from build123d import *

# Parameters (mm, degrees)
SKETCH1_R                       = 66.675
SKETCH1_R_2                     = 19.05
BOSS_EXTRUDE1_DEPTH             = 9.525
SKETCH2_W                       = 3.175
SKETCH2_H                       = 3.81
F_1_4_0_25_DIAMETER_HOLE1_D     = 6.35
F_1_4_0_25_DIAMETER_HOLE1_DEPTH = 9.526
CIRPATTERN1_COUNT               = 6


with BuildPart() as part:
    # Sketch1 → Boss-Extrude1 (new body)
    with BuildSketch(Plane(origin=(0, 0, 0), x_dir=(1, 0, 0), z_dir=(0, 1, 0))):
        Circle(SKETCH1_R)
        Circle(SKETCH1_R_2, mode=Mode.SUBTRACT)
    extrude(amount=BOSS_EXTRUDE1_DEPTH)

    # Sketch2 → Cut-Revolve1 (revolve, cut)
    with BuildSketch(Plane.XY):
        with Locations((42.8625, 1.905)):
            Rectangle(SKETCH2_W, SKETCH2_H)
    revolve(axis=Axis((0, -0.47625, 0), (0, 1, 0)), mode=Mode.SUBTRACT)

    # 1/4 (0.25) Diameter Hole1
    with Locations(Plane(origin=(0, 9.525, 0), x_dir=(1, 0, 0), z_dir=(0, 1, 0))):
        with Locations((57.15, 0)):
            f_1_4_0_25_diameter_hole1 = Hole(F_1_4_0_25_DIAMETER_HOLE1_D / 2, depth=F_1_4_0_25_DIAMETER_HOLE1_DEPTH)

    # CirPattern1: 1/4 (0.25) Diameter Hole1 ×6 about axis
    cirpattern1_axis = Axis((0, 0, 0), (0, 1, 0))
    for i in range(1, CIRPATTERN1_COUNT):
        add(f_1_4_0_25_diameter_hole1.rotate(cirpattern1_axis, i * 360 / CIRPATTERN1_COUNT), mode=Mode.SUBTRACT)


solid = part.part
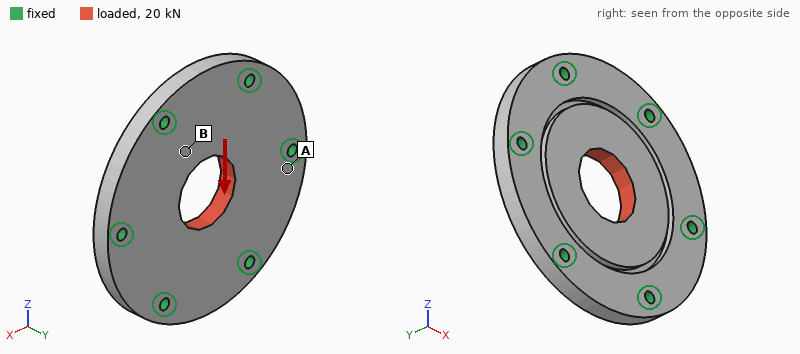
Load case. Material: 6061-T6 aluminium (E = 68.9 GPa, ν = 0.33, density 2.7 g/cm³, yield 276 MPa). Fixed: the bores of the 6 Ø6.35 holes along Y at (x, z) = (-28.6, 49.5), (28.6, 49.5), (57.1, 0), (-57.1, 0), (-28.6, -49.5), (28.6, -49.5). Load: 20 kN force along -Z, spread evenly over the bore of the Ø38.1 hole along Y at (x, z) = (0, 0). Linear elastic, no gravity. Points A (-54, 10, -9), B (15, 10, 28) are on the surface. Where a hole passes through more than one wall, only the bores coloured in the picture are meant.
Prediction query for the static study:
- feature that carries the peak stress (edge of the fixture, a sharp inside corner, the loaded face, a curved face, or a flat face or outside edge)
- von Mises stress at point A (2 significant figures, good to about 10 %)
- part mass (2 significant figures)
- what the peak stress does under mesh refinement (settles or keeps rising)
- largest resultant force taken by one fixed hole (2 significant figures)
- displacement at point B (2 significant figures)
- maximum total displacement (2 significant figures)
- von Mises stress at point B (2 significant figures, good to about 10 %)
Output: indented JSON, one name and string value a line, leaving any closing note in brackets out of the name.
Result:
{
  "feature that carries the peak stress": "edge of the fixture",
  "von Mises stress at point A": "7.9 MPa",
  "part mass": "320 g",
  "what the peak stress does under mesh refinement": "keeps rising",
  "largest resultant force taken by one fixed hole": "4.2 kN",
  "displacement at point B": "8.9 µm",
  "maximum total displacement": "15 µm",
  "von Mises stress at point B": "18 MPa"
}
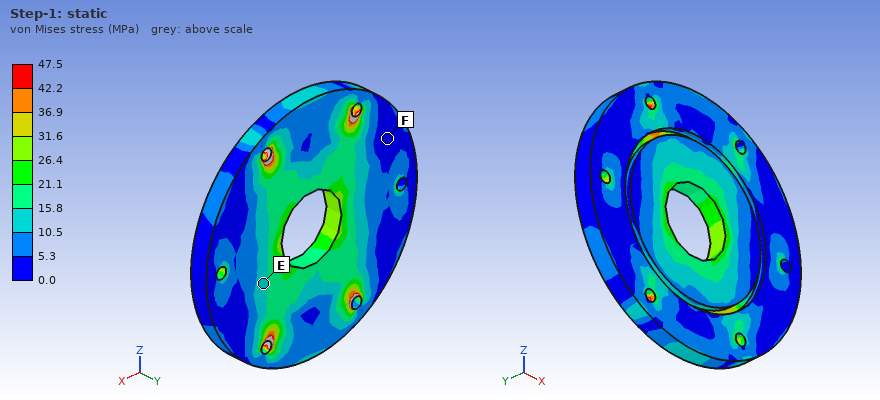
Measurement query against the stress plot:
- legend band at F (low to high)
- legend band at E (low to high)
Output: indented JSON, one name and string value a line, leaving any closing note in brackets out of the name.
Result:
{
  "legend band at F": "0.0 to 5.3 MPa",
  "legend band at E": "10.5 to 15.8 MPa"
}
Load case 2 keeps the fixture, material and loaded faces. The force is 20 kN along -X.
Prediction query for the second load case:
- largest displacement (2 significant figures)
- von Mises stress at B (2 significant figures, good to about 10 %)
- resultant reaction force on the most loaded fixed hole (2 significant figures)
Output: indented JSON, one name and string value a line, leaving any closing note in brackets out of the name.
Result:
{
  "largest displacement": "15 µm",
  "von Mises stress at B": "15 MPa",
  "resultant reaction force on the most loaded fixed hole": "4.7 kN"
}
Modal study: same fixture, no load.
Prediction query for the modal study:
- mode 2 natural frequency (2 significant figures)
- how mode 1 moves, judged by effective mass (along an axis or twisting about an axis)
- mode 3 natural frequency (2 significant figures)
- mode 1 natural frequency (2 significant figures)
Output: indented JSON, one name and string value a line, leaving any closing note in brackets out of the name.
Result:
{
  "mode 2 natural frequency": "9700 Hz",
  "how mode 1 moves, judged by effective mass": "along Y",
  "mode 3 natural frequency": "9700 Hz",
  "mode 1 natural frequency": "6000 Hz"
}
